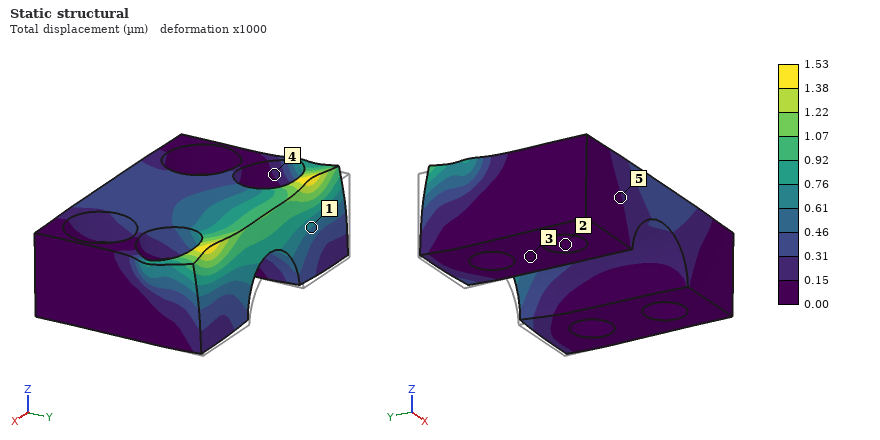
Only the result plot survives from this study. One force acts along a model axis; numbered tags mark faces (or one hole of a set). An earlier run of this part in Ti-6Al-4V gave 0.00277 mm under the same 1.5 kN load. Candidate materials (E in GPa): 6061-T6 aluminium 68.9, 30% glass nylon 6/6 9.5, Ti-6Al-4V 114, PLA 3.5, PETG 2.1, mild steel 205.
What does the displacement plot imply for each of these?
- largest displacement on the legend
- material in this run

1.53 µm
mild steel
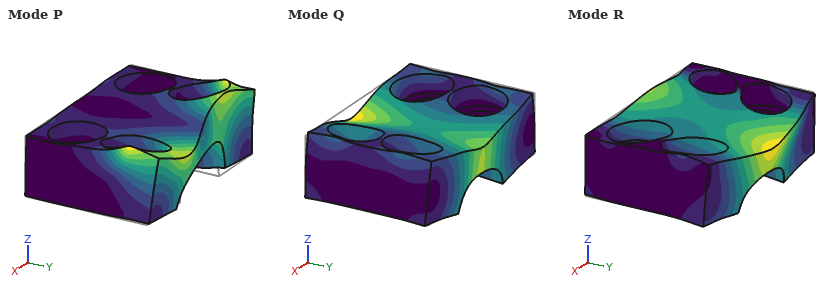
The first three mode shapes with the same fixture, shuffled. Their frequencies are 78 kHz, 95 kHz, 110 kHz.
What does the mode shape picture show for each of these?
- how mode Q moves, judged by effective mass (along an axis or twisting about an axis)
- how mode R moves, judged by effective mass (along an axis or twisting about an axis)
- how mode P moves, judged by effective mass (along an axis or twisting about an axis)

along Z
along Y
along X
